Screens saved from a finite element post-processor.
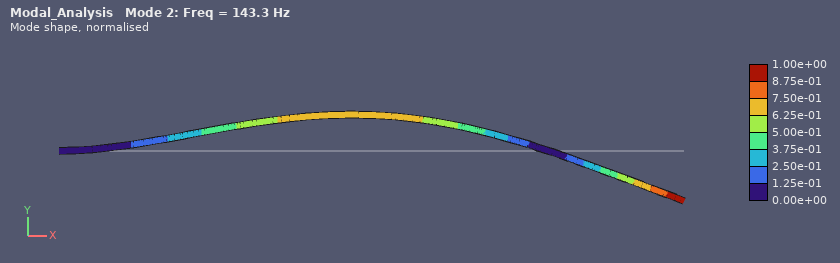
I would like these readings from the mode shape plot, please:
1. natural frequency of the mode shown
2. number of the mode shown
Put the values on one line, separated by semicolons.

143.3 Hz; 2
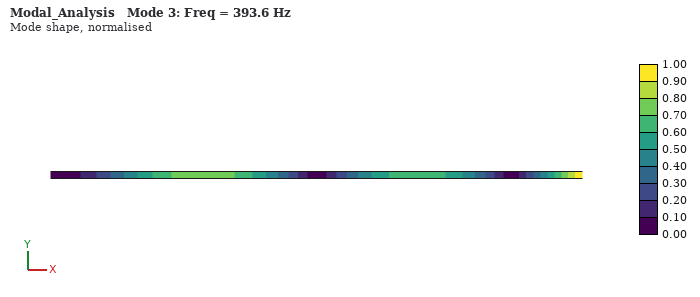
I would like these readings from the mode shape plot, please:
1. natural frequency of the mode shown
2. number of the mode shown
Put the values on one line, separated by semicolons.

393.6 Hz; 3
